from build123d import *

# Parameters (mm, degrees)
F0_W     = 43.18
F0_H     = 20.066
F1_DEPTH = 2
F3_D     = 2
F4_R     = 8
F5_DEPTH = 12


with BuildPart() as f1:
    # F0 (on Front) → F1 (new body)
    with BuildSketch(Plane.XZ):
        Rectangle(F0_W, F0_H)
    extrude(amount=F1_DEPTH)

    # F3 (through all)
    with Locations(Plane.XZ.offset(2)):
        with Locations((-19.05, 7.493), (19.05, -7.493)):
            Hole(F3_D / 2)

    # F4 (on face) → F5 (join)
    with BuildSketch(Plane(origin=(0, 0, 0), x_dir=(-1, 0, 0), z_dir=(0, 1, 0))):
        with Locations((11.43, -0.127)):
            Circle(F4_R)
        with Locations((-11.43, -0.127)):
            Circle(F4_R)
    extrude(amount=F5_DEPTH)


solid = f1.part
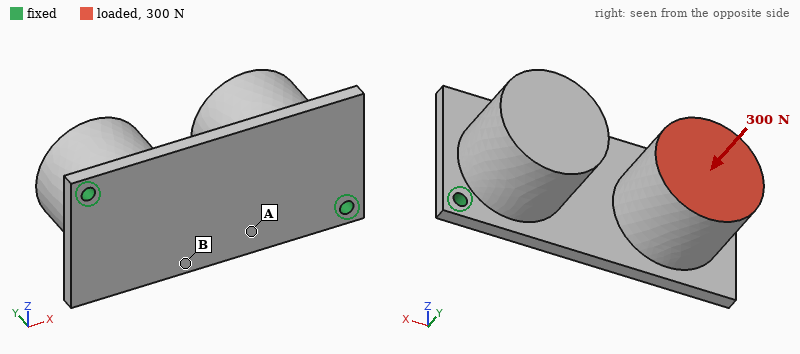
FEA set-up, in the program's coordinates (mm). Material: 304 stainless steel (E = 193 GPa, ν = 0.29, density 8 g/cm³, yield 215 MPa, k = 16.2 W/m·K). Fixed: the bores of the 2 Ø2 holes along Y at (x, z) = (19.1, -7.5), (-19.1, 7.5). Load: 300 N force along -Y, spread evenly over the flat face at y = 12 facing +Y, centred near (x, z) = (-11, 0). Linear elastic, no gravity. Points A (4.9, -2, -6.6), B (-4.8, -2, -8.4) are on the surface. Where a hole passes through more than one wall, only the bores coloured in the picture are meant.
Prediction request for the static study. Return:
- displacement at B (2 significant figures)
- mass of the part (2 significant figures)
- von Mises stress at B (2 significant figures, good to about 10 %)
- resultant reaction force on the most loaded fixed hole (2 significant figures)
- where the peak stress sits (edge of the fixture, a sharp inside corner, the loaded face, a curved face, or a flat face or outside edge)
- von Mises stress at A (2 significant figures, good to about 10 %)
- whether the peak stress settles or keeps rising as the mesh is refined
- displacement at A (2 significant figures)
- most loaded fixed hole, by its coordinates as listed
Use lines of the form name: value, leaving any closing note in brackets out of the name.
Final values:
displacement at B: 36 µm
mass of the part: 52 g
von Mises stress at B: 64 MPa
resultant reaction force on the most loaded fixed hole: 230 N
where the peak stress sits: edge of the fixture
von Mises stress at A: 22 MPa
whether the peak stress settles or keeps rising as the mesh is refined: keeps rising
displacement at A: 20 µm
most loaded fixed hole, by its coordinates as listed: (-19.1, 7.5)
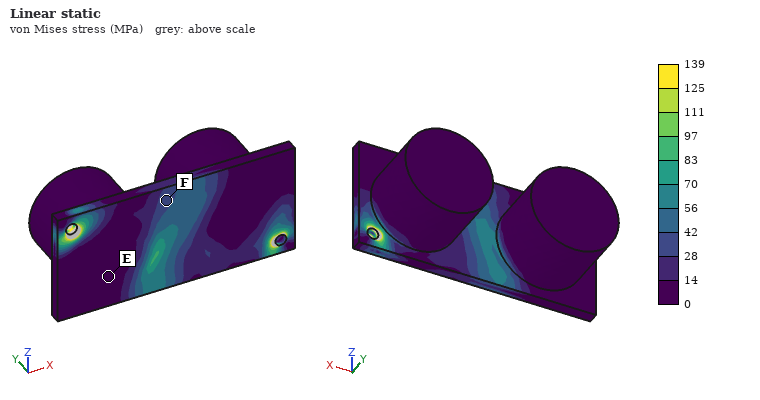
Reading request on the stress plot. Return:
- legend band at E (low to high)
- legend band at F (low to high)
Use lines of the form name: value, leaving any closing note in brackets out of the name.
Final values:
legend band at E: 0 to 14 MPa
legend band at F: 28 to 42 MPa
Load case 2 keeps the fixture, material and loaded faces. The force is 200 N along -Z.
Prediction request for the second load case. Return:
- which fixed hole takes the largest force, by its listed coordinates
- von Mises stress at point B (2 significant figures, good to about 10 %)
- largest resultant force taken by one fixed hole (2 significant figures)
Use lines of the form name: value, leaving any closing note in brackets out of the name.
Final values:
which fixed hole takes the largest force, by its listed coordinates: (-19.1, 7.5)
von Mises stress at point B: 47 MPa
largest resultant force taken by one fixed hole: 160 N
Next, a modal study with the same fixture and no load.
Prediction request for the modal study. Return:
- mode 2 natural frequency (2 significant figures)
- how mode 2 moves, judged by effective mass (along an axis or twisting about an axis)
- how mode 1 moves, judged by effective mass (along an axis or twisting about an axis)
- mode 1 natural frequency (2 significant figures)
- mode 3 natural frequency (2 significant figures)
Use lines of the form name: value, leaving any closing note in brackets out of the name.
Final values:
mode 2 natural frequency: 2600 Hz
how mode 2 moves, judged by effective mass: along Y
how mode 1 moves, judged by effective mass: along Z
mode 1 natural frequency: 2400 Hz
mode 3 natural frequency: 4700 Hz
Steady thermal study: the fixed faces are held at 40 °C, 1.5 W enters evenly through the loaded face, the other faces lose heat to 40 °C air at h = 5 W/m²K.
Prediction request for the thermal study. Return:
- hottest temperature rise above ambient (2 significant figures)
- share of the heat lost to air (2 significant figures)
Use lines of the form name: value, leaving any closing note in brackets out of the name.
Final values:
hottest temperature rise above ambient: 22 K
share of the heat lost to air: 12 %
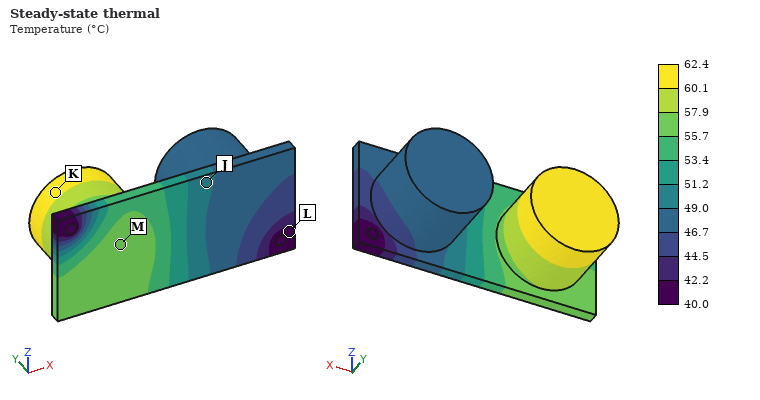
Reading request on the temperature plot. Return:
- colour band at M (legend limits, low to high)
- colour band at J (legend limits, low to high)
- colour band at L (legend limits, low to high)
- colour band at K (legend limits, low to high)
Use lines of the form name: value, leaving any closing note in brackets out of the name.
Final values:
colour band at M: 55.7 to 57.9 °C
colour band at J: 49.0 to 51.2 °C
colour band at L: 40.0 to 42.2 °C
colour band at K: 60.1 to 62.4 °C
